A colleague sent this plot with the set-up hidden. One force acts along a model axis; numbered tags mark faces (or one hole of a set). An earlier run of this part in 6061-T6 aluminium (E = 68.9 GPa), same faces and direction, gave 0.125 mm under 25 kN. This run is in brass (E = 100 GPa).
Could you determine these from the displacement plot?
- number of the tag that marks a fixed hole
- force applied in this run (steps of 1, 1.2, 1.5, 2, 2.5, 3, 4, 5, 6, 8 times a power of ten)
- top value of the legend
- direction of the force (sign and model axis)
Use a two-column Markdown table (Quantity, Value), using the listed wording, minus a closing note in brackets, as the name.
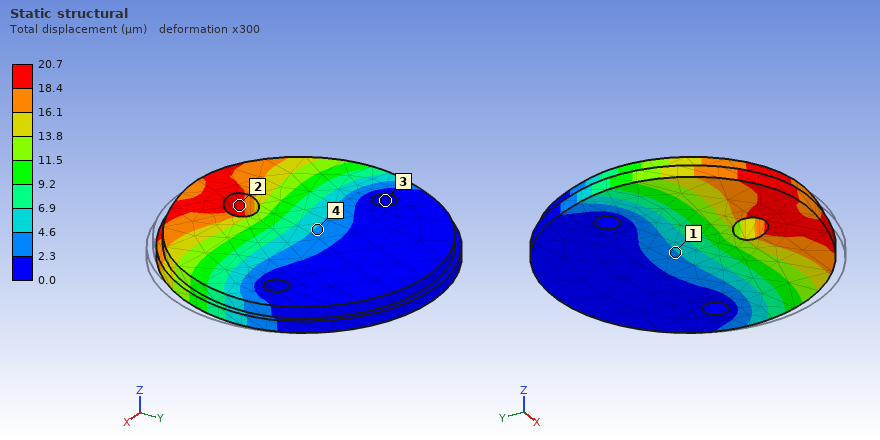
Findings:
| Quantity | Value |
|---|---|
| number of the tag that marks a fixed hole | 3 |
| force applied in this run | 6 kN |
| top value of the legend | 20.7 µm |
| direction of the force | -X |
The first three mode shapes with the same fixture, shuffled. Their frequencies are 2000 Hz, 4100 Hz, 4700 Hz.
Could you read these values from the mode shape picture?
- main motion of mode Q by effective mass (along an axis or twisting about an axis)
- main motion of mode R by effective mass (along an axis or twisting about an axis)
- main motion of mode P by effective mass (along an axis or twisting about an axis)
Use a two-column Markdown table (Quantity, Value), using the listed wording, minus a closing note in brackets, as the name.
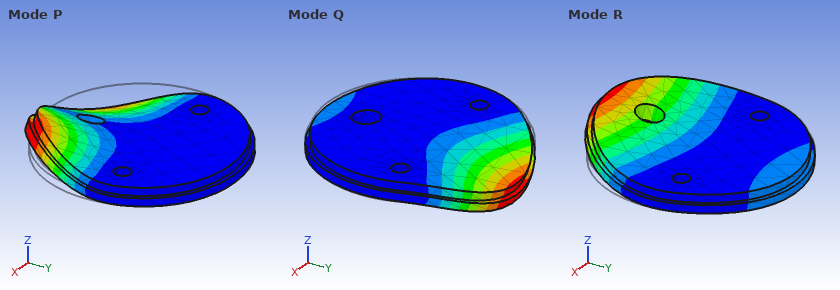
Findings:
| Quantity | Value |
|---|---|
| main motion of mode Q by effective mass | along Z |
| main motion of mode R by effective mass | along Z |
| main motion of mode P by effective mass | twisting about Y |
